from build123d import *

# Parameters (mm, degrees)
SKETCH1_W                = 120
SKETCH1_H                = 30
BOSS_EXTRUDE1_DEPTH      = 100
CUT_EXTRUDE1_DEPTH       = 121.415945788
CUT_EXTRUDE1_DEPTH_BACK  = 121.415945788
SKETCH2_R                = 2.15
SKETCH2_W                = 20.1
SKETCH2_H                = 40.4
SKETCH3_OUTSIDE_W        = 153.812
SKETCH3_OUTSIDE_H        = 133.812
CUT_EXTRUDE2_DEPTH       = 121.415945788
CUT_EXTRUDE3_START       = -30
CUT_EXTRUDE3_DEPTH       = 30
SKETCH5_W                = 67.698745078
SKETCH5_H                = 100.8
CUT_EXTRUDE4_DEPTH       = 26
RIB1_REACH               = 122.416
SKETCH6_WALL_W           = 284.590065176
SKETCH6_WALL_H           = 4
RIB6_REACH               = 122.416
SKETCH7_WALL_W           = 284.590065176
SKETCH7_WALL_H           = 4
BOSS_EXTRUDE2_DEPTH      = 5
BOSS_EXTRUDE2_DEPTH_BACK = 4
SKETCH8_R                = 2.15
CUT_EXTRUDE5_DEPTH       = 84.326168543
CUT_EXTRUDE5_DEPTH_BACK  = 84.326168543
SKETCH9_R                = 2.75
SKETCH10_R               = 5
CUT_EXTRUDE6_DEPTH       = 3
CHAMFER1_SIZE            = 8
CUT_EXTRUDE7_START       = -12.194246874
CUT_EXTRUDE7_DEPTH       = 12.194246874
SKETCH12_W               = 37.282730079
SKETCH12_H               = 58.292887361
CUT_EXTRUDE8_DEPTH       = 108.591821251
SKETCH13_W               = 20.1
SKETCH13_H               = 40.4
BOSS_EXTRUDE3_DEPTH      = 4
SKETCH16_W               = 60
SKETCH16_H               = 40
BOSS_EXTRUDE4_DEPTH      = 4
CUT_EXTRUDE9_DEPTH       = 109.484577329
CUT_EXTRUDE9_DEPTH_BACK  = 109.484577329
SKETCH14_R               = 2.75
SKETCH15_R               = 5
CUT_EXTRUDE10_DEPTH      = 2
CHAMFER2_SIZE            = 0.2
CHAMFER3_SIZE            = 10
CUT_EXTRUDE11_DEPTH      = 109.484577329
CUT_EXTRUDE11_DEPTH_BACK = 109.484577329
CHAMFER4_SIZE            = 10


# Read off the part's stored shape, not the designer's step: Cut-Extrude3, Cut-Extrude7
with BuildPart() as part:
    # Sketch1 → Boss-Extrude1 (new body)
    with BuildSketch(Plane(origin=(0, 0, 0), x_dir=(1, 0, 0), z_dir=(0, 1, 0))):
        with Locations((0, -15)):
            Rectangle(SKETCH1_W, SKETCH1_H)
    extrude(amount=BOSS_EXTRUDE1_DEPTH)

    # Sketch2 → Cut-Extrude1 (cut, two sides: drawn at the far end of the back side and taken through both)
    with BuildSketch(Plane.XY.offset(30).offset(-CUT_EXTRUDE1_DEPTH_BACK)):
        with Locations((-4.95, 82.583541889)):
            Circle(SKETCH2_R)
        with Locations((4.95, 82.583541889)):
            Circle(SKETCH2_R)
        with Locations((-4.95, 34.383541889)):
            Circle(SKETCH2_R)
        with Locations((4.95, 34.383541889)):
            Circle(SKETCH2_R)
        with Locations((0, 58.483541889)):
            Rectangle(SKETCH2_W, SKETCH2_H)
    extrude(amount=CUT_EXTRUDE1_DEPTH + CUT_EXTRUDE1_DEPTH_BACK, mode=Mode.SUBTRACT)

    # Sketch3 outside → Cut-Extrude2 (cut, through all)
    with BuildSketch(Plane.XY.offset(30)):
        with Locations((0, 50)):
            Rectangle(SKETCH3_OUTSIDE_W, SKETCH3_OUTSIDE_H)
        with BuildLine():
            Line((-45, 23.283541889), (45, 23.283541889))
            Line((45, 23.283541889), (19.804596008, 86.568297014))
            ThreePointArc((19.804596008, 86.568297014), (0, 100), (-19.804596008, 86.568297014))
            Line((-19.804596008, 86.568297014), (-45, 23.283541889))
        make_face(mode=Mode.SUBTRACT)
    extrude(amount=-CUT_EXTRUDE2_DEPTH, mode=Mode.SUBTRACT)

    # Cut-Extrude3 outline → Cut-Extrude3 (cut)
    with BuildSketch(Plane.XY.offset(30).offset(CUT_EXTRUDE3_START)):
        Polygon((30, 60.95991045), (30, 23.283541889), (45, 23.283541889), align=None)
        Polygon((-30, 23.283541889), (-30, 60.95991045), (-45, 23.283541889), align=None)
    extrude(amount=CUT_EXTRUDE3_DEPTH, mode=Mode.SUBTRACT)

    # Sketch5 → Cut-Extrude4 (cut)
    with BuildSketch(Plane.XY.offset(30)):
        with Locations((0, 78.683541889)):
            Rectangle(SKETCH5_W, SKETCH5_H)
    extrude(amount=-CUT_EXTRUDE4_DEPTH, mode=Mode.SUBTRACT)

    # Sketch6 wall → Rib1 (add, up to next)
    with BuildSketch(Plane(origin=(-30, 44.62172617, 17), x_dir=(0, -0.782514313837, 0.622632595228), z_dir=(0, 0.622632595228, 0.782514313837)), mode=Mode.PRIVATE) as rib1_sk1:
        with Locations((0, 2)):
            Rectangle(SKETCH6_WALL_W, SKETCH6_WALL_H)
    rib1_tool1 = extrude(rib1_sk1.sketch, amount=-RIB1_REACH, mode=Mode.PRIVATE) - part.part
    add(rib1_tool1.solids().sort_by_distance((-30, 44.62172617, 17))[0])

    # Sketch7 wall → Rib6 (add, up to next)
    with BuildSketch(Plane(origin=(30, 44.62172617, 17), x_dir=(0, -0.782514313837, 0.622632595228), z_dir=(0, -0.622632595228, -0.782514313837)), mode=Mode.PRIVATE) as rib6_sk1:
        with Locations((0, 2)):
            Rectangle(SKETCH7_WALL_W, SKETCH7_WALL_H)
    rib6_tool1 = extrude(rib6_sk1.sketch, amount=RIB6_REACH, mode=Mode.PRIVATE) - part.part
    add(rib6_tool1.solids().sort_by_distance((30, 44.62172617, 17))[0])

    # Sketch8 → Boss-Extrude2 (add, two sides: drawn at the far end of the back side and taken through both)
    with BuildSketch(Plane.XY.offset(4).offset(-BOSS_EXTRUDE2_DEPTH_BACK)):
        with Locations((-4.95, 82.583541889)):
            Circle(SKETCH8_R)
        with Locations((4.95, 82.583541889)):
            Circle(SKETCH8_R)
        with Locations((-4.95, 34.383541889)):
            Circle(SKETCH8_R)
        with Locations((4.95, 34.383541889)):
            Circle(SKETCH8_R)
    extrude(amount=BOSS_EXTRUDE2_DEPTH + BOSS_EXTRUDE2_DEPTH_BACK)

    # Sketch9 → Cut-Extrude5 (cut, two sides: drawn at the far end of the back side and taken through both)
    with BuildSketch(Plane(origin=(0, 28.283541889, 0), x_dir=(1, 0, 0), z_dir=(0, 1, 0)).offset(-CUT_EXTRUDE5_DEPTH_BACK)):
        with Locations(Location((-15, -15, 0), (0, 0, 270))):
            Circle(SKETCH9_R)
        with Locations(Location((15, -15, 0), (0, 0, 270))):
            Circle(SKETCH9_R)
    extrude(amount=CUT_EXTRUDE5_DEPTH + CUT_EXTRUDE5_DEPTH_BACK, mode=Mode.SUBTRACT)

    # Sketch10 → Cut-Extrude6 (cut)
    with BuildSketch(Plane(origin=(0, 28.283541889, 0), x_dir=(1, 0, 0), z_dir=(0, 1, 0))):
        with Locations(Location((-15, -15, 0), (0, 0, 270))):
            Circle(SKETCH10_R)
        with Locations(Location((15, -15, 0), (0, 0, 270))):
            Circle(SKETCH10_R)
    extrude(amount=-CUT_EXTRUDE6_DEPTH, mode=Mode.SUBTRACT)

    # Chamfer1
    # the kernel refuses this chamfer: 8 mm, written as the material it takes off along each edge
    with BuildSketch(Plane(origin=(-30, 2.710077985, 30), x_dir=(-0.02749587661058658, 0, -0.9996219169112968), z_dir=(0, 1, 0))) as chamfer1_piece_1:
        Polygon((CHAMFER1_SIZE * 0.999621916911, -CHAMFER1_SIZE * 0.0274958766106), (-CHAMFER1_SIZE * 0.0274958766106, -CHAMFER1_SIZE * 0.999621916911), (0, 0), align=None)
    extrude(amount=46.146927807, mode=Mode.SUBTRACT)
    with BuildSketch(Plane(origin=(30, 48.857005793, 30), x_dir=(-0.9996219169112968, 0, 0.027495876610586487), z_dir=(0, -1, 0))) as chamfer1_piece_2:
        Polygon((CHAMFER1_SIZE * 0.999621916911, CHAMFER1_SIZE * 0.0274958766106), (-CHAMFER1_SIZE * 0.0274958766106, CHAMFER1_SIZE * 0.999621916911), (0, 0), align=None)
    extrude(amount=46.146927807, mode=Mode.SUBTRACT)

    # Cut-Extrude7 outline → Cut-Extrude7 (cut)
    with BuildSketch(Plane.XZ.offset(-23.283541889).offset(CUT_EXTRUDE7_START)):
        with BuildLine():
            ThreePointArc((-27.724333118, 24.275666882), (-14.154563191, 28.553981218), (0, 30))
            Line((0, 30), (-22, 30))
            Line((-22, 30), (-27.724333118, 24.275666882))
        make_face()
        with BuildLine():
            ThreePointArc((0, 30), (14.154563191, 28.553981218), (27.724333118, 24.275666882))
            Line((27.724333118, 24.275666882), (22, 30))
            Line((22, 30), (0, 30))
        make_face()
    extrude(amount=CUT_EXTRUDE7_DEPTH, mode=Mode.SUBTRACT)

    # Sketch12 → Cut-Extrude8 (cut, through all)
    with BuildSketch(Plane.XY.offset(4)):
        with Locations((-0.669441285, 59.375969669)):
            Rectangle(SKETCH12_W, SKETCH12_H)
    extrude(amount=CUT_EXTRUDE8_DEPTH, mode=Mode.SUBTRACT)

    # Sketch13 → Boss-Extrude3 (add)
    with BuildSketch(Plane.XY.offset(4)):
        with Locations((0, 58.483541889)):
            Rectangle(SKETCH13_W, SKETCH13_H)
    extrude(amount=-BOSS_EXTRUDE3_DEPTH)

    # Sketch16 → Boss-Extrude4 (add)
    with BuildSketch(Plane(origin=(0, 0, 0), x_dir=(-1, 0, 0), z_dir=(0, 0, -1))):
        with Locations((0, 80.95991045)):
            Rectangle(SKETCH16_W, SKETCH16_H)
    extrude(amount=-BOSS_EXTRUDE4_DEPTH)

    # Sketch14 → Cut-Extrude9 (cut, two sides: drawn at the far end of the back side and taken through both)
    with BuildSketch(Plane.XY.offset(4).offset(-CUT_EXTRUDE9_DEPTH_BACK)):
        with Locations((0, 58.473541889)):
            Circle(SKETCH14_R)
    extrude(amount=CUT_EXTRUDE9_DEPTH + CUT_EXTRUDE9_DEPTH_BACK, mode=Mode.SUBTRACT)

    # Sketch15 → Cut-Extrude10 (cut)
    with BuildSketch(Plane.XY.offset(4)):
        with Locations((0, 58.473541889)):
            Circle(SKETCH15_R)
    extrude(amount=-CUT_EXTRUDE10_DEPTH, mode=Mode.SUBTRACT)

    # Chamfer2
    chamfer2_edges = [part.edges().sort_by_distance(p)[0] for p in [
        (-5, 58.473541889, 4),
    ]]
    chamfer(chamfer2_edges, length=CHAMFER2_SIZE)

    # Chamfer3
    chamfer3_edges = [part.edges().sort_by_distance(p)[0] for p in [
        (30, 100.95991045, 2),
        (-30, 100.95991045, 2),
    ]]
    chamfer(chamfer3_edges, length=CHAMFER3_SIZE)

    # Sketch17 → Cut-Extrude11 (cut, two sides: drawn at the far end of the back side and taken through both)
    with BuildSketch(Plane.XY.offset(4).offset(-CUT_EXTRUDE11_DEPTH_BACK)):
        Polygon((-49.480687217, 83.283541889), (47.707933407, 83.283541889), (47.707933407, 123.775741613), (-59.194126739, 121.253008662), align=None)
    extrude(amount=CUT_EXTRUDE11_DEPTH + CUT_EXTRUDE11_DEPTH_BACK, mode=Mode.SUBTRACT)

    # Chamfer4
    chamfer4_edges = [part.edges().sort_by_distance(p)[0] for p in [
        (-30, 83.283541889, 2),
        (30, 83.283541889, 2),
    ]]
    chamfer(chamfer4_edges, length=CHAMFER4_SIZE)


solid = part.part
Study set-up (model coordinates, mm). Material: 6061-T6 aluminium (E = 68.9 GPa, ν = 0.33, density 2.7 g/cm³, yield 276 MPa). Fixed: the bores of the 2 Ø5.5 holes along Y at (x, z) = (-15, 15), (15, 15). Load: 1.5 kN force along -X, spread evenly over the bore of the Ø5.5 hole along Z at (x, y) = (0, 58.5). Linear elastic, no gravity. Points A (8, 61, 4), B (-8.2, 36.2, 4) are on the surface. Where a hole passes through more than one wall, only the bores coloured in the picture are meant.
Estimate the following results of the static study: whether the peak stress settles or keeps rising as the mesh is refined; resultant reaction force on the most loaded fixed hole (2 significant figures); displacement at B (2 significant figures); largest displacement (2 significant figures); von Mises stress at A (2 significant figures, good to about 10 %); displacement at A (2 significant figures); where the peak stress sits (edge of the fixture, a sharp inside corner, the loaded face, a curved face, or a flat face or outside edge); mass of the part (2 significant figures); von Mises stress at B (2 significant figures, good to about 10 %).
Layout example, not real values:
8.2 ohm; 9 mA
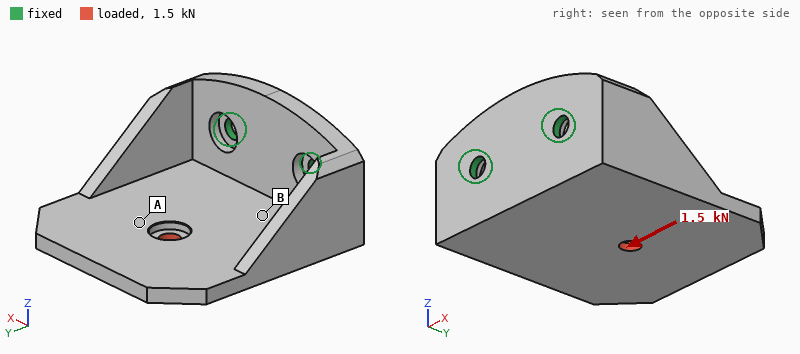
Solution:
keeps rising; 1.9 kN; 0.055 mm; 0.26 mm; 21 MPa; 0.15 mm; edge of the fixture; 64 g; 41 MPa
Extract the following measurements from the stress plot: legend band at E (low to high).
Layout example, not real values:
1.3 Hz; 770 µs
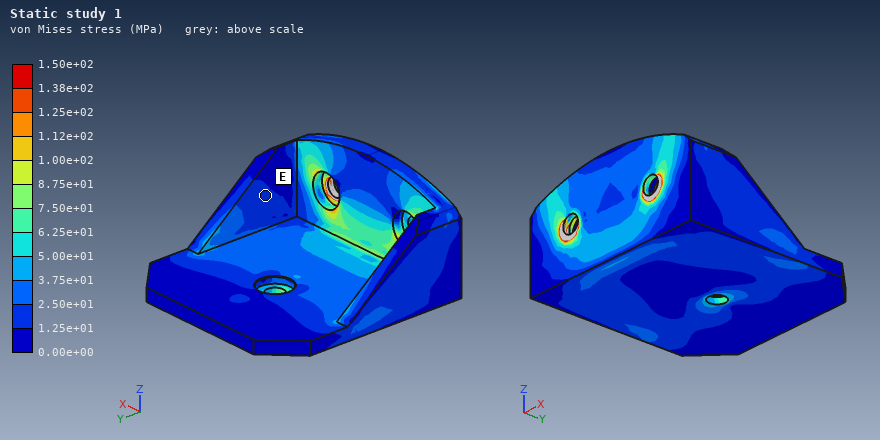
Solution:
1.25e+01 to 2.50e+01 MPa
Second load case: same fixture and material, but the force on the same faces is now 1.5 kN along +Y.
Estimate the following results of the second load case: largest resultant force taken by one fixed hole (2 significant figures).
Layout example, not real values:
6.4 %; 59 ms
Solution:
760 N
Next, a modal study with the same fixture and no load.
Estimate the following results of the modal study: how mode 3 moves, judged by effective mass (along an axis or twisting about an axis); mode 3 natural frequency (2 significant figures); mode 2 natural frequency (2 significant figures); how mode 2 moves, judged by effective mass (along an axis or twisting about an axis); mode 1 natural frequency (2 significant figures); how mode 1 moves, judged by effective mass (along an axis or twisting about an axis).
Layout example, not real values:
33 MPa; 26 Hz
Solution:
along X; 4200 Hz; 2100 Hz; along X; 1000 Hz; along Z
